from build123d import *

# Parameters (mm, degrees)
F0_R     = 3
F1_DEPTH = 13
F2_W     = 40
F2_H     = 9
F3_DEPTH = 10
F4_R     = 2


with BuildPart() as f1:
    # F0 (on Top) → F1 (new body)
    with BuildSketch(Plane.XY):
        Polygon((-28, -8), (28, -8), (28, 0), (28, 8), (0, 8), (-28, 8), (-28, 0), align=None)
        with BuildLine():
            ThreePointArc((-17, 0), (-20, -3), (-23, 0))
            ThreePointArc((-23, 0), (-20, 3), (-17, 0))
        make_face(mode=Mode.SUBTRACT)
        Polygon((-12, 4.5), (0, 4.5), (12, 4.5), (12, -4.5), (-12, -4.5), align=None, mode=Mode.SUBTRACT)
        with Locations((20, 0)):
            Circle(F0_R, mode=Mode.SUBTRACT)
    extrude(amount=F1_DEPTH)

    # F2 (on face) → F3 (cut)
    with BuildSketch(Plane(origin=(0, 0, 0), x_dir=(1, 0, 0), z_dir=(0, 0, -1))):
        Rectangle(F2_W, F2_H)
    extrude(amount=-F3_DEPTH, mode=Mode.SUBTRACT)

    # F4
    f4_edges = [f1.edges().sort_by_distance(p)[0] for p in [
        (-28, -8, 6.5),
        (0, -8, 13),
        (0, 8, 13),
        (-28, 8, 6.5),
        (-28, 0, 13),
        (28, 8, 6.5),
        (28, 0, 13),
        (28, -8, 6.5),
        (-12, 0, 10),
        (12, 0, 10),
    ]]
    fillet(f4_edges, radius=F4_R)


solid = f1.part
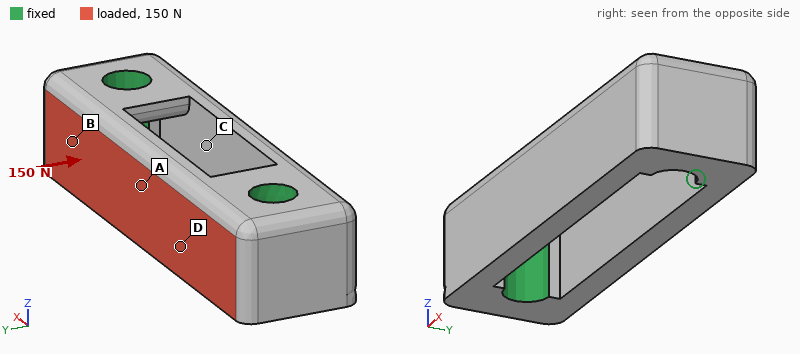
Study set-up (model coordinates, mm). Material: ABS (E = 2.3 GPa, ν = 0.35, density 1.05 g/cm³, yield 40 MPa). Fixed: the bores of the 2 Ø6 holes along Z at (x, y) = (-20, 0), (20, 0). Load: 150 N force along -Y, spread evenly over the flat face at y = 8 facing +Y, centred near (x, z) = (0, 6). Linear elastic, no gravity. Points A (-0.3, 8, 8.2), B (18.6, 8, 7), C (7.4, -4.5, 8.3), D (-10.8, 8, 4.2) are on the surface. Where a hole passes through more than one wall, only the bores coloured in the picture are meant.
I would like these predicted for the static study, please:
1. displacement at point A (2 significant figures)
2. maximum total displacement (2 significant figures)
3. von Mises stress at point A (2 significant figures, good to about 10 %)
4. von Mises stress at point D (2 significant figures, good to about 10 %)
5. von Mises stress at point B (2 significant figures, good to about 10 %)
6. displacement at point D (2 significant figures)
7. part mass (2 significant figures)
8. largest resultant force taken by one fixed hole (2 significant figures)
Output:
0.13 mm
0.22 mm
6.2 MPa
3.4 MPa
5.7 MPa
0.096 mm
7.1 g
79 N
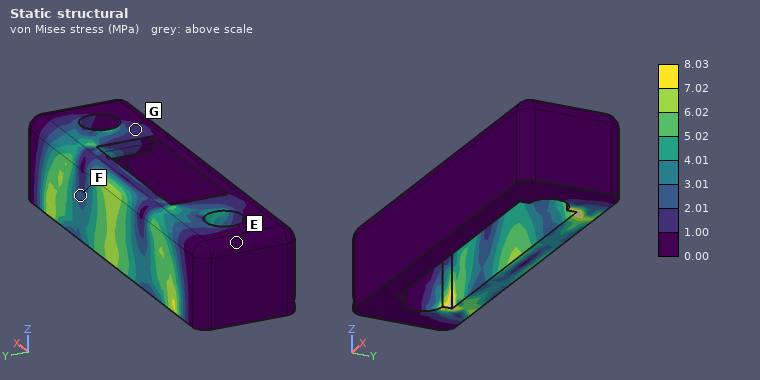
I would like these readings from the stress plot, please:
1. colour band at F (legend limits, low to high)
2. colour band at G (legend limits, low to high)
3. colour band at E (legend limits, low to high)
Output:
2.01 to 3.01 MPa
1.00 to 2.01 MPa
0.00 to 1.00 MPa
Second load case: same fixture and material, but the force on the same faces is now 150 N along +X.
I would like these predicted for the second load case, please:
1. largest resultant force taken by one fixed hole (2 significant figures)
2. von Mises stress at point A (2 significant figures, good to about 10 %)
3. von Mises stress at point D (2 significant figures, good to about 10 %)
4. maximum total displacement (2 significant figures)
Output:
76 N
0.56 MPa
0.47 MPa
13 µm
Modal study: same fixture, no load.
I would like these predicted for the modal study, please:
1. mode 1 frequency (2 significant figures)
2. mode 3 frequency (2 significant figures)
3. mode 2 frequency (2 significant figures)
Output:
3600 Hz
6800 Hz
3700 Hz
